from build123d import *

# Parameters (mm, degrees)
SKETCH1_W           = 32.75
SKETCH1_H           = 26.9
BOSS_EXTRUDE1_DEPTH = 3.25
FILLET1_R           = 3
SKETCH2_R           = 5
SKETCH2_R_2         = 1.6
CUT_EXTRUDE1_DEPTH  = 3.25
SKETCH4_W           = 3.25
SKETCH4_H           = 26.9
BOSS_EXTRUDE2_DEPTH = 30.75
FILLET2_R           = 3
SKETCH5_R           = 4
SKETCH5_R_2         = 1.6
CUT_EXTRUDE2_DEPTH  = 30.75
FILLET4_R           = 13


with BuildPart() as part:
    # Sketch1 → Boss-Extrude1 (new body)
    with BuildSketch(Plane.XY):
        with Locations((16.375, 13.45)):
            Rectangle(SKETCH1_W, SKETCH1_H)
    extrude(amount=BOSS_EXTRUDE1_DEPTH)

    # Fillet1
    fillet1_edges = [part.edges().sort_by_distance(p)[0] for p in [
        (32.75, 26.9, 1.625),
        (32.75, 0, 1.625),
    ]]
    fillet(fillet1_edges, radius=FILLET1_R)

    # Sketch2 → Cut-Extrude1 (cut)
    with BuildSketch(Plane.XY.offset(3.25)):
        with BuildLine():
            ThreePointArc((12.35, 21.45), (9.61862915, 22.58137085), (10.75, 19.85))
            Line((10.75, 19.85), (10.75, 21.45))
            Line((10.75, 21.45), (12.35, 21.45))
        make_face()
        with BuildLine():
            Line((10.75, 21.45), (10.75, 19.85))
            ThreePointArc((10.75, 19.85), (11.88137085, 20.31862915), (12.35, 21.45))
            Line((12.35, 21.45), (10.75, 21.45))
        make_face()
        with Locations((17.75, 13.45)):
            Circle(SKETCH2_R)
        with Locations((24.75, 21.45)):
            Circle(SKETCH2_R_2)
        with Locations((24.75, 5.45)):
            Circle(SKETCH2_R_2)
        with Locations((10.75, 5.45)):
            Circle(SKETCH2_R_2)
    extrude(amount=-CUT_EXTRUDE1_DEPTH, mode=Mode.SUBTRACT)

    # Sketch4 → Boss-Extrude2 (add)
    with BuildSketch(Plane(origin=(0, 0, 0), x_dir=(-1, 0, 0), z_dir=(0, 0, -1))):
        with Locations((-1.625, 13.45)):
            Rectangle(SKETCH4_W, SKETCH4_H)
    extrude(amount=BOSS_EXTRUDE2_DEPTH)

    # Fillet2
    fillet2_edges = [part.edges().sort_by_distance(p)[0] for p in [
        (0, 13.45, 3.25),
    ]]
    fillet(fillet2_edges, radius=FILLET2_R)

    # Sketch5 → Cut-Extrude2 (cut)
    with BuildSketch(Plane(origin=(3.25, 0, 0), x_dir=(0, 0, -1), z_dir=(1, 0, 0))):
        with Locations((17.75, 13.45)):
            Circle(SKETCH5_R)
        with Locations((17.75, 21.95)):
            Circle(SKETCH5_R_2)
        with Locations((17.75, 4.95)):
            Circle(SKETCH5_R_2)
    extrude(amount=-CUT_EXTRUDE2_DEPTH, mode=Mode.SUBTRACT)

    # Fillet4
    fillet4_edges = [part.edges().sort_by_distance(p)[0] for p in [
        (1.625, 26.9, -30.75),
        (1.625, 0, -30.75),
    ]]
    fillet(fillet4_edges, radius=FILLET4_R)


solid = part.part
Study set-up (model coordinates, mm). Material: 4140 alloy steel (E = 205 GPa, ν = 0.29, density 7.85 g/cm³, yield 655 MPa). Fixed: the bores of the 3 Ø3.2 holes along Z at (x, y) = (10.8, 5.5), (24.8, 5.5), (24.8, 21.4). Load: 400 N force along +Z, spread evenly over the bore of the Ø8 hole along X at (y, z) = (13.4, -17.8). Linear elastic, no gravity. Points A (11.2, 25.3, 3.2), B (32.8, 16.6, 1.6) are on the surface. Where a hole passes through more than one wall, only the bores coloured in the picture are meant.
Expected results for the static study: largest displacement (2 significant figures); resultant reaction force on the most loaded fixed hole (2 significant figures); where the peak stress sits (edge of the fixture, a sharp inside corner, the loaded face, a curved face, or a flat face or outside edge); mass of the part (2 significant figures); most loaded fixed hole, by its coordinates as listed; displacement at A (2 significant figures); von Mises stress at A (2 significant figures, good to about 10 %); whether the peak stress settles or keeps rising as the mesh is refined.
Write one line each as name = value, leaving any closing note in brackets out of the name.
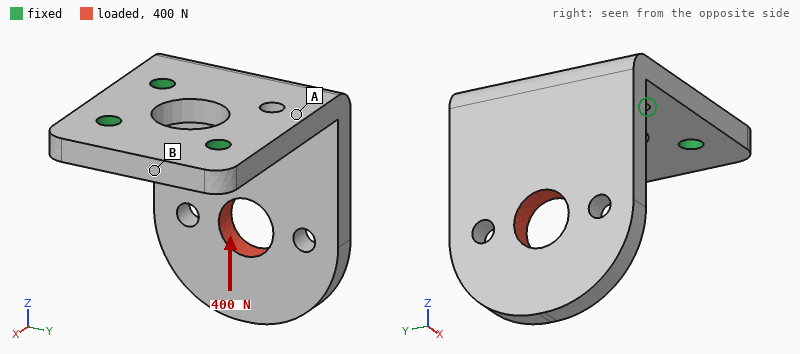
largest displacement = 79 µm
resultant reaction force on the most loaded fixed hole = 400 N
where the peak stress sits = edge of the fixture
mass of the part = 37 g
most loaded fixed hole, by its coordinates as listed = (10.8, 5.5)
displacement at A = 15 µm
von Mises stress at A = 40 MPa
whether the peak stress settles or keeps rising as the mesh is refined = keeps rising
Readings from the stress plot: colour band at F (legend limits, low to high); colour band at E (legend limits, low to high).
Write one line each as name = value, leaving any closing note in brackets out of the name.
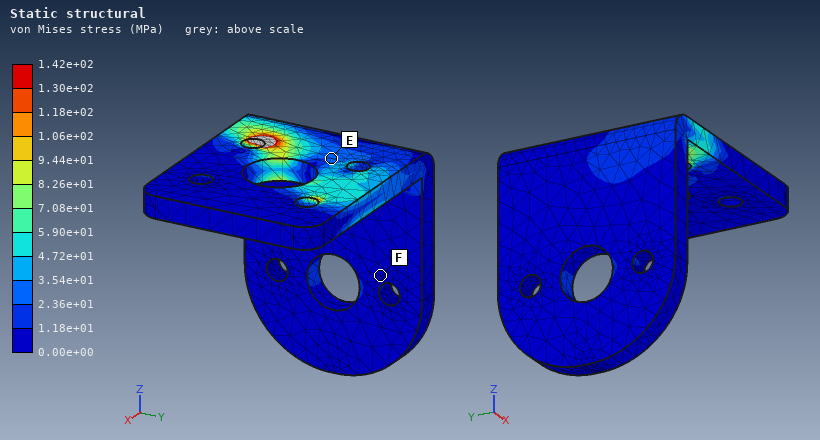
colour band at F = 0.00e+00 to 1.18e+01 MPa
colour band at E = 2.36e+01 to 3.54e+01 MPa
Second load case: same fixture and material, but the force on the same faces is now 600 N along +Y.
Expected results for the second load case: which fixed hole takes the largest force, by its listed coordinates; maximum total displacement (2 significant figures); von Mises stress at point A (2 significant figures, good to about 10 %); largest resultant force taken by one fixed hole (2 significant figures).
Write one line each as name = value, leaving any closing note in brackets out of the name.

which fixed hole takes the largest force, by its listed coordinates = (10.8, 5.5)
maximum total displacement = 0.18 mm
von Mises stress at point A = 97 MPa
largest resultant force taken by one fixed hole = 660 N
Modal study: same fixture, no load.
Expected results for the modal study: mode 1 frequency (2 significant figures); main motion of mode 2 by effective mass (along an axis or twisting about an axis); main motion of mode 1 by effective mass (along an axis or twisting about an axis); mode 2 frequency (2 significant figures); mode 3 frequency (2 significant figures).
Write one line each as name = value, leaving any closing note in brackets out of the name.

mode 1 frequency = 1900 Hz
main motion of mode 2 by effective mass = along Y
main motion of mode 1 by effective mass = along X
mode 2 frequency = 3100 Hz
mode 3 frequency = 7400 Hz
